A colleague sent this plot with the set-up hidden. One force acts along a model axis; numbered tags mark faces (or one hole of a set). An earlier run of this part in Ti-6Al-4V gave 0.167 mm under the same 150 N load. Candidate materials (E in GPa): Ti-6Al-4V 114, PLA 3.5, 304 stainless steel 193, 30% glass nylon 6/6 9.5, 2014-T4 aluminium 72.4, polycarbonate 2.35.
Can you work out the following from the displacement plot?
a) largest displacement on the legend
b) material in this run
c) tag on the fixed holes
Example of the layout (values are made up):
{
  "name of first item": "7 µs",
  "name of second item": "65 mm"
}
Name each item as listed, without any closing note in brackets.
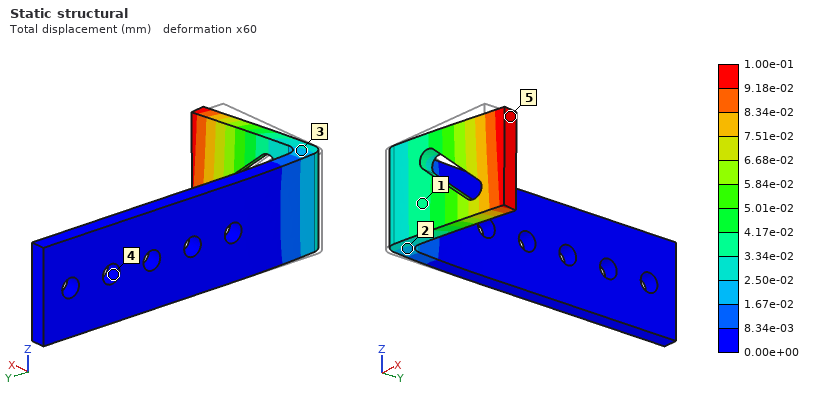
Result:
{
  "largest displacement on the legend": "1.00e-01 mm",
  "material in this run": "304 stainless steel",
  "tag on the fixed holes": "4"
}
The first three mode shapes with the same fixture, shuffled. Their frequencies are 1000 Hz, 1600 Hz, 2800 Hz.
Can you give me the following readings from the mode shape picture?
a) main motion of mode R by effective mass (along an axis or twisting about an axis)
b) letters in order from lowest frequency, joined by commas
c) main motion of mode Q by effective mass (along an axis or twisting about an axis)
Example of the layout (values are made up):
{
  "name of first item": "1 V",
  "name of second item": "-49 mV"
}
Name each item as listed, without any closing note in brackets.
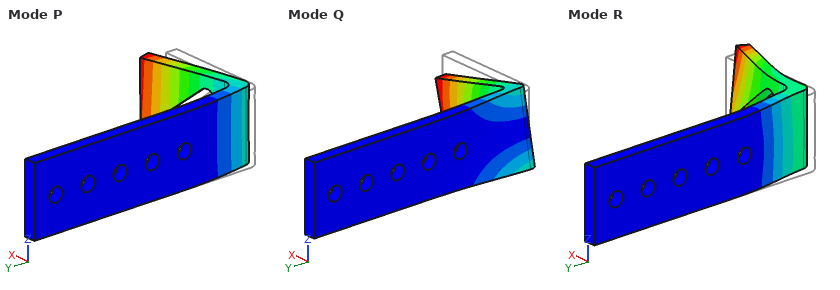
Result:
{
  "main motion of mode R by effective mass": "along X",
  "letters in order from lowest frequency, joined by commas": "P, Q, R",
  "main motion of mode Q by effective mass": "along Z"
}
